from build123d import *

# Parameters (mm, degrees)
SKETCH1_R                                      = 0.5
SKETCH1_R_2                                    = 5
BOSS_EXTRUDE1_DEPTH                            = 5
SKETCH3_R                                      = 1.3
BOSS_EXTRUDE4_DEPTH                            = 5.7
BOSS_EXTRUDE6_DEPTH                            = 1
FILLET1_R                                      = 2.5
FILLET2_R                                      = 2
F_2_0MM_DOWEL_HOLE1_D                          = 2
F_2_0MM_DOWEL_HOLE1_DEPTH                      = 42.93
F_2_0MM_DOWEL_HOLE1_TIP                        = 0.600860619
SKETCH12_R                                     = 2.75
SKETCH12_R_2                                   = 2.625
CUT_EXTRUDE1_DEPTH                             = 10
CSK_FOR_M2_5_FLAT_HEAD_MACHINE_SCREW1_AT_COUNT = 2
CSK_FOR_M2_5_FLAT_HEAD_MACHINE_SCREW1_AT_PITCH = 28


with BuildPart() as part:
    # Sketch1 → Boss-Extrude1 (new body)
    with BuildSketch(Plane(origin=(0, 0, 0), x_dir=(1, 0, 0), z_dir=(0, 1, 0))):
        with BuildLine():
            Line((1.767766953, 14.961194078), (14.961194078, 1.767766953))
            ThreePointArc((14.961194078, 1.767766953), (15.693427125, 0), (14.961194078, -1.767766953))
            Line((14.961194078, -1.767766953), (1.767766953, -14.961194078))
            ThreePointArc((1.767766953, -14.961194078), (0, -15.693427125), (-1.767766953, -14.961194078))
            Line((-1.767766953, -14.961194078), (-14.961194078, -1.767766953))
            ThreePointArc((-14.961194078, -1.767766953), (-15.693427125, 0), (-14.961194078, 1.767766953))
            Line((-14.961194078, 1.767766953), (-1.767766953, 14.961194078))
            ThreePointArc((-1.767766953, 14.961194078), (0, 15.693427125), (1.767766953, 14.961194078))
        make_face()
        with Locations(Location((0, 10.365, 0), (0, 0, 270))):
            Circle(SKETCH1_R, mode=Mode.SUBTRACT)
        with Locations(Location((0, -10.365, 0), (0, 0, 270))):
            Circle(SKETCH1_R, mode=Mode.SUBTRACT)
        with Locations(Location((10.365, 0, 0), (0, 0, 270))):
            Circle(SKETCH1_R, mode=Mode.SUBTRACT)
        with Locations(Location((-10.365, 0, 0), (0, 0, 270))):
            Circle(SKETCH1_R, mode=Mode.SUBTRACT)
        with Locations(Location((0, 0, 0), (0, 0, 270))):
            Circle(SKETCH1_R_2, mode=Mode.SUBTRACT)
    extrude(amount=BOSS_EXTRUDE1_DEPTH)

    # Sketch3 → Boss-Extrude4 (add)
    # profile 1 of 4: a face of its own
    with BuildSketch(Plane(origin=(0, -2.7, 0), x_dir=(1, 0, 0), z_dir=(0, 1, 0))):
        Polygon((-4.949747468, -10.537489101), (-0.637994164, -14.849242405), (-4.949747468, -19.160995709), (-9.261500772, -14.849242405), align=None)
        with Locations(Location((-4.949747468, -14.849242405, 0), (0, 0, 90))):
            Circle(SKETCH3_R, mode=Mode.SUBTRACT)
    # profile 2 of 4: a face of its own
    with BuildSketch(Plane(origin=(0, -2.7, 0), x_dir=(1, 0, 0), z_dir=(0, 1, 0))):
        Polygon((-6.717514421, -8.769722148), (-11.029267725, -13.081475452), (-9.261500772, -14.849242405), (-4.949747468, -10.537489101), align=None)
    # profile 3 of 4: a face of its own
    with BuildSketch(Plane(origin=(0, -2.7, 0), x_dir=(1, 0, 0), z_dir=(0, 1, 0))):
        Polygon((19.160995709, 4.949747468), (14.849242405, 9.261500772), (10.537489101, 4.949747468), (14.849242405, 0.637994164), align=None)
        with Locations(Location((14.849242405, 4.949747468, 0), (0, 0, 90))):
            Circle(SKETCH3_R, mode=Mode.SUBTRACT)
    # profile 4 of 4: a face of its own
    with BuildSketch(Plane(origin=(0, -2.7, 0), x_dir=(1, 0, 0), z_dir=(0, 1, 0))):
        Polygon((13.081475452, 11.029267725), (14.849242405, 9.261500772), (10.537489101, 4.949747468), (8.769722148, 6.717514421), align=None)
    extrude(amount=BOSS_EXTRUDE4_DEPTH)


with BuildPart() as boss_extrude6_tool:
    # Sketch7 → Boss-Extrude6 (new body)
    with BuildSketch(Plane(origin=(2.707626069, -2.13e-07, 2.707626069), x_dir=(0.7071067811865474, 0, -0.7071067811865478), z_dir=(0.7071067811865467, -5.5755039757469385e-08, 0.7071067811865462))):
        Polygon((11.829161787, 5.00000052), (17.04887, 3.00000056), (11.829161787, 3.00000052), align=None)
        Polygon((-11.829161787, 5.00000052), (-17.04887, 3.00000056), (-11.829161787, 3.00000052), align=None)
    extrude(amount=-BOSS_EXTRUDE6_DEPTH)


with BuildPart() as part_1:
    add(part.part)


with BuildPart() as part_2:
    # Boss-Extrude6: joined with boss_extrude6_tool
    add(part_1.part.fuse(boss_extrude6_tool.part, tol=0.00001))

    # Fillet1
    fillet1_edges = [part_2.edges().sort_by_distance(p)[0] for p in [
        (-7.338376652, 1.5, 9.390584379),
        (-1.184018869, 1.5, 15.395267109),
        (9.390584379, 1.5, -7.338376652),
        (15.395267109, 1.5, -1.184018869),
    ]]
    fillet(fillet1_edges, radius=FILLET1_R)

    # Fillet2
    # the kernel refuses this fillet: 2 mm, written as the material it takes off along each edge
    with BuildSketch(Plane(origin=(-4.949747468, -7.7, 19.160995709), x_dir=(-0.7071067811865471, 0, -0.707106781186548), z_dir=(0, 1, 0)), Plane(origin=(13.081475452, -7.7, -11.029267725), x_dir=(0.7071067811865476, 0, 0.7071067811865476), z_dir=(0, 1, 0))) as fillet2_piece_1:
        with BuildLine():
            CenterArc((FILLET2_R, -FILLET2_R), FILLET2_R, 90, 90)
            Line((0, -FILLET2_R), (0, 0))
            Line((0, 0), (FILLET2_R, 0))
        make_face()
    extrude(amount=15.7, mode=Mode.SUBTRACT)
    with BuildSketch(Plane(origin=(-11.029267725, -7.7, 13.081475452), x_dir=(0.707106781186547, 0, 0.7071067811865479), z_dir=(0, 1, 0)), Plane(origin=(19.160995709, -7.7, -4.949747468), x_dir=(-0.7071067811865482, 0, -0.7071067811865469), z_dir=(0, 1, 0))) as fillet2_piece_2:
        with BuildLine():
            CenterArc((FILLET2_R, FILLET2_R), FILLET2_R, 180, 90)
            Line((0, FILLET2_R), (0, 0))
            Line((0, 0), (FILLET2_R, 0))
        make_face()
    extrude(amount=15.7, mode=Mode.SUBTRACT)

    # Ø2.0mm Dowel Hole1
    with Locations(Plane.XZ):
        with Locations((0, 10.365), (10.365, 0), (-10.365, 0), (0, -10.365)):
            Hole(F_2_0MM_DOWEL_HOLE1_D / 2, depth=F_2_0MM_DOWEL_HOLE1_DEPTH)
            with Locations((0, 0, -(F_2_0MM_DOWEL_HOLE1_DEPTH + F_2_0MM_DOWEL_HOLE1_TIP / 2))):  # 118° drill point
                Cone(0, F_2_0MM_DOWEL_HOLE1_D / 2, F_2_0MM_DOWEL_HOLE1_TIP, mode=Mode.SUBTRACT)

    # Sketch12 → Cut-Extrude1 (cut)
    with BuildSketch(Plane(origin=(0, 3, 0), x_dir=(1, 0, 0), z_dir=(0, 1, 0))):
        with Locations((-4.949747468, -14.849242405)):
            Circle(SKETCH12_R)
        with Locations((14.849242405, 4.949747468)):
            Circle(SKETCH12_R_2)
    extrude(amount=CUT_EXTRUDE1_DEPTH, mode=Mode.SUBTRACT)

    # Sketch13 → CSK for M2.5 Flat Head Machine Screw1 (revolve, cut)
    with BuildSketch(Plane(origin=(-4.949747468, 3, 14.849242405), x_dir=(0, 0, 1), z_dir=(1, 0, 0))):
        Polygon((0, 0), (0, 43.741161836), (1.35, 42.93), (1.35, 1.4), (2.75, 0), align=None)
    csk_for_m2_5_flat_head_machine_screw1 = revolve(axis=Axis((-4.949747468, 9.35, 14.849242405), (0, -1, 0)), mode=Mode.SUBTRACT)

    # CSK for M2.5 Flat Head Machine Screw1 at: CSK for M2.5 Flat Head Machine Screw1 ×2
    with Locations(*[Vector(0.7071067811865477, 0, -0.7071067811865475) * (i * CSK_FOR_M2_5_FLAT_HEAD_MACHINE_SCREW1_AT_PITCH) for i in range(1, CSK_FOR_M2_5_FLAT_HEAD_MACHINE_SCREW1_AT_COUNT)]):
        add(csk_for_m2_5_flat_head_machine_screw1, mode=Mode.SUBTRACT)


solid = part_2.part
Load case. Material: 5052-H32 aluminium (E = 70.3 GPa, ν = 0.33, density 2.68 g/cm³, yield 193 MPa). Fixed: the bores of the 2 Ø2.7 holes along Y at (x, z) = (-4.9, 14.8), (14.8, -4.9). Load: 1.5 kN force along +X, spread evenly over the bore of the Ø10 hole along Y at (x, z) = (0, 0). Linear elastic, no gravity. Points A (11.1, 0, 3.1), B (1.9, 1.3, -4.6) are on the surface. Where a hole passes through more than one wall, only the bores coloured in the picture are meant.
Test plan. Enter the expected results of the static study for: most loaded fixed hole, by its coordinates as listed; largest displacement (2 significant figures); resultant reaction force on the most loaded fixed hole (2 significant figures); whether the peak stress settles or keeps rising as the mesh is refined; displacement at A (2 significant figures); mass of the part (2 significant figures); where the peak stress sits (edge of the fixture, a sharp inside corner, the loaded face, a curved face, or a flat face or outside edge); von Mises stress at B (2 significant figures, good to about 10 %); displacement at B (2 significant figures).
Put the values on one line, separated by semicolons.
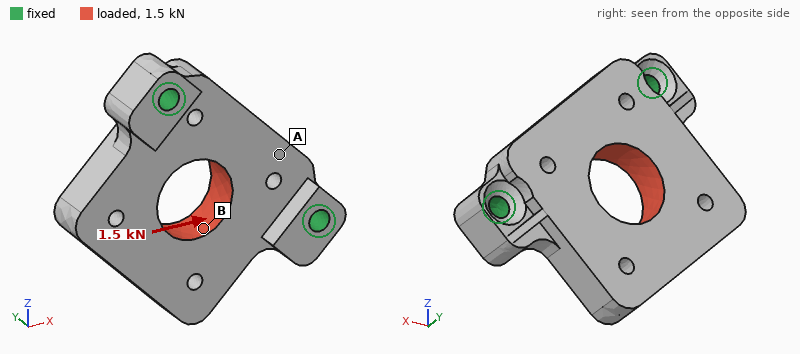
(14.8, -4.9); 25 µm; 980 N; keeps rising; 5.8 µm; 7.4 g; edge of the fixture; 33 MPa; 13 µm
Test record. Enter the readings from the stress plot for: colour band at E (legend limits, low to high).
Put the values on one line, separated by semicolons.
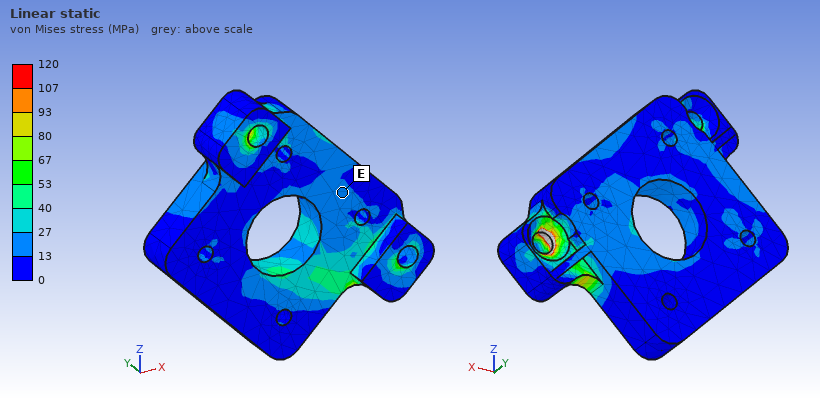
13 to 27 MPa
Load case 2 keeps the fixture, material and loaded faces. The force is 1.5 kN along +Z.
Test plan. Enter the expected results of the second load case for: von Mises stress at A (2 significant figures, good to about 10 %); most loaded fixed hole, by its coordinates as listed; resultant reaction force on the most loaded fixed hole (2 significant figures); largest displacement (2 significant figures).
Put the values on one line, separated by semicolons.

24 MPa; (-4.9, 14.8); 990 N; 25 µm
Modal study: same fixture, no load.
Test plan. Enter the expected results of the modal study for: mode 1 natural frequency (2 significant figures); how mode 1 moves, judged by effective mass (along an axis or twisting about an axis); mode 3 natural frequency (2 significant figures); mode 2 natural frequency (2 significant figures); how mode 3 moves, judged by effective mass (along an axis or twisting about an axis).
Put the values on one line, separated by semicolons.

7600 Hz; along Y; 26 kHz; 19 kHz; along Y
